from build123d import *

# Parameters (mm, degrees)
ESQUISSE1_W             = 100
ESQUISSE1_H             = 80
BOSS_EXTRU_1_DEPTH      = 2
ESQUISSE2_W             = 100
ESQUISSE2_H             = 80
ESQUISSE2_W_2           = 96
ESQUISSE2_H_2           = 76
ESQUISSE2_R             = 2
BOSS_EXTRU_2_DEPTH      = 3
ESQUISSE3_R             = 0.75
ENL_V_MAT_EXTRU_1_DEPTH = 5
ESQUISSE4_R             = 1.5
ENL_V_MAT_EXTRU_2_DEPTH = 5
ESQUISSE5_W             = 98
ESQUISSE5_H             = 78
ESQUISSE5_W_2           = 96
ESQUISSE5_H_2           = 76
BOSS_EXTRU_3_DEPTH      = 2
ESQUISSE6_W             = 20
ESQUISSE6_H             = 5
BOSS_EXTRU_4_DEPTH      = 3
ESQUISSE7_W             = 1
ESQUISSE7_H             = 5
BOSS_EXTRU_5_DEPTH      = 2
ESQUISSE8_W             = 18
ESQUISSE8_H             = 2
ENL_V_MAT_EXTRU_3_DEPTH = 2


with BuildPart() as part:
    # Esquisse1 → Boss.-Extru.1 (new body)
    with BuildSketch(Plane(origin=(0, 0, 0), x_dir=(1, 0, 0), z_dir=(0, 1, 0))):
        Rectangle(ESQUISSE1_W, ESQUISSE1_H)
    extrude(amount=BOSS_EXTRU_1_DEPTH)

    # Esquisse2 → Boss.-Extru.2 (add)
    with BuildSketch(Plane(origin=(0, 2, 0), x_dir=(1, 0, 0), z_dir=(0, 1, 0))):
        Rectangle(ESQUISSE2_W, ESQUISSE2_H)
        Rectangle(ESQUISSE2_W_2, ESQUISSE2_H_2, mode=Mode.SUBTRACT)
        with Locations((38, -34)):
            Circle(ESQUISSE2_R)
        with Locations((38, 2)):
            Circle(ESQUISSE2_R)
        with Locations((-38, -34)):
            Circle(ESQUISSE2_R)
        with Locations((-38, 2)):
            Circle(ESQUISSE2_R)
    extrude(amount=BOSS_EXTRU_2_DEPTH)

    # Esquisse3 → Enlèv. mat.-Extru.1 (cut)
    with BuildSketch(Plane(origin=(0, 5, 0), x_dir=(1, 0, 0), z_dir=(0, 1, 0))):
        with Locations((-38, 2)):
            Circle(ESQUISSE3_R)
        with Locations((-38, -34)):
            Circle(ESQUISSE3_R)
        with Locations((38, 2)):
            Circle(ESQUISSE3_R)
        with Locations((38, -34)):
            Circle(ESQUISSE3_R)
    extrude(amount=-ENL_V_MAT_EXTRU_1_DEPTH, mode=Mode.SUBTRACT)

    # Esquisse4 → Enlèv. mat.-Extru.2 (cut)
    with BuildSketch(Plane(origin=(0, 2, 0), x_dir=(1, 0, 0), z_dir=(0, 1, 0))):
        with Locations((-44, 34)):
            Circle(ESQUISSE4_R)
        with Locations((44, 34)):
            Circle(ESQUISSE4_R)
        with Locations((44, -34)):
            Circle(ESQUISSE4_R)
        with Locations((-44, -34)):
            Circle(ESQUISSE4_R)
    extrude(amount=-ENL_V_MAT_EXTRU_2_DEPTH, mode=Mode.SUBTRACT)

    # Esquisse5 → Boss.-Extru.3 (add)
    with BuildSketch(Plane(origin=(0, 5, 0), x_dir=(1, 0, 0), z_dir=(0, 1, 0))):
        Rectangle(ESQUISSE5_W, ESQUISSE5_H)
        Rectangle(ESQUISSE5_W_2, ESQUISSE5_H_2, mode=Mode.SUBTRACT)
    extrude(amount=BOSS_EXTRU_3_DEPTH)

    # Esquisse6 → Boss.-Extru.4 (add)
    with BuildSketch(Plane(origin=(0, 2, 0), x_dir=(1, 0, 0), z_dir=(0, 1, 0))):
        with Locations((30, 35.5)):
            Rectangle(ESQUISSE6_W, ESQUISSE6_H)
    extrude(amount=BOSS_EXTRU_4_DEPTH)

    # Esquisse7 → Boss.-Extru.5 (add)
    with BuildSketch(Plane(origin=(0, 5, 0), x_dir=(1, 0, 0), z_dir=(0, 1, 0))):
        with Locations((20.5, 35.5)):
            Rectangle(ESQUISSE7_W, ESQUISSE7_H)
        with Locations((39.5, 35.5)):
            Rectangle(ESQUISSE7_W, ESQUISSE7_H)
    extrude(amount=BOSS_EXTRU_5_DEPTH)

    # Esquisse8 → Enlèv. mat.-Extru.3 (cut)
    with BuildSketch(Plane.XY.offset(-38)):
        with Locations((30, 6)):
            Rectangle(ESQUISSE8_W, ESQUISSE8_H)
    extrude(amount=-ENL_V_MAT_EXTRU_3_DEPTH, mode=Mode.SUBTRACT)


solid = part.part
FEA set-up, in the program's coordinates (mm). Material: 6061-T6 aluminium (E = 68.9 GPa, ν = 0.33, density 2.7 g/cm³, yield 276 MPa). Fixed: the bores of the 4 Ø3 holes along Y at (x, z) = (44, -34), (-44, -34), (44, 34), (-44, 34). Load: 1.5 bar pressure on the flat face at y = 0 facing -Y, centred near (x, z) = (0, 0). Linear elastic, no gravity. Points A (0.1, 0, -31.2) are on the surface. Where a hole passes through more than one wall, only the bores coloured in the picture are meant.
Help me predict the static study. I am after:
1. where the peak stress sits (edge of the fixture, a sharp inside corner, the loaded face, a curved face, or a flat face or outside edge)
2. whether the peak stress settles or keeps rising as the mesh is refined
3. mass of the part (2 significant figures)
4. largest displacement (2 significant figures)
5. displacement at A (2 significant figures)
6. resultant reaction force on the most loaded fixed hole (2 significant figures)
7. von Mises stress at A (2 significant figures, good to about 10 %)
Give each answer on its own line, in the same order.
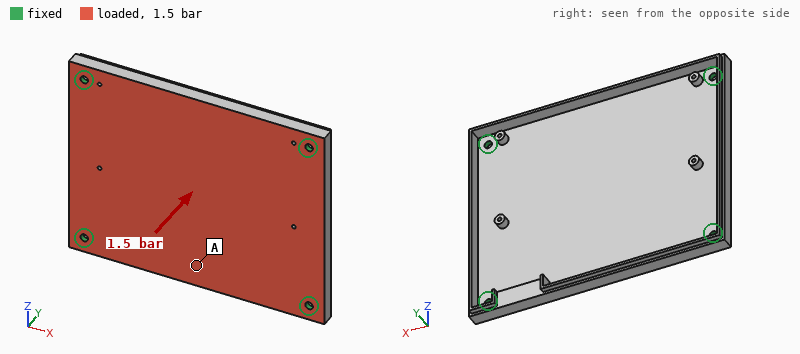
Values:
edge of the fixture
keeps rising
52 g
0.58 mm
0.31 mm
320 N
41 MPa
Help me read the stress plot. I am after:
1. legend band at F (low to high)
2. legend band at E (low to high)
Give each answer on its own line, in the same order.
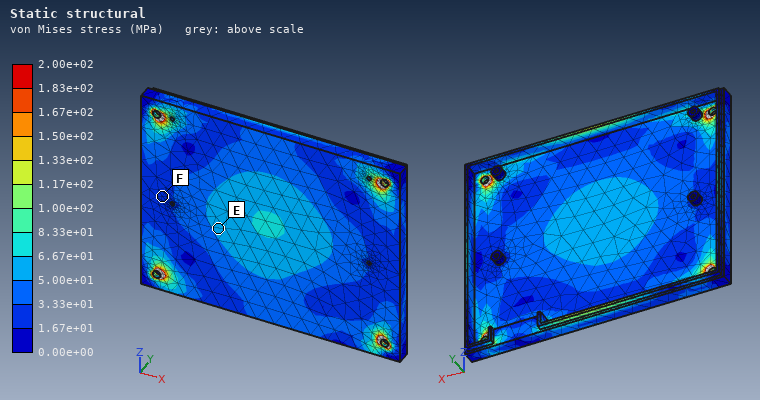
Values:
1.67e+01 to 3.33e+01 MPa
5.00e+01 to 6.67e+01 MPa
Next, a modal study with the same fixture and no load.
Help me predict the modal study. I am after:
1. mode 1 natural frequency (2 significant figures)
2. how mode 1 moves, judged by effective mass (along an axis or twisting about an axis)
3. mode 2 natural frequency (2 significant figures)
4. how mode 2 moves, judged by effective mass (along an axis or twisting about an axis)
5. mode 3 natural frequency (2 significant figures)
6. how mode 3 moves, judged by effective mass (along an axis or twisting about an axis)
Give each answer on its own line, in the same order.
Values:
1400 Hz
along Y
2400 Hz
twisting about X
2800 Hz
twisting about Z
